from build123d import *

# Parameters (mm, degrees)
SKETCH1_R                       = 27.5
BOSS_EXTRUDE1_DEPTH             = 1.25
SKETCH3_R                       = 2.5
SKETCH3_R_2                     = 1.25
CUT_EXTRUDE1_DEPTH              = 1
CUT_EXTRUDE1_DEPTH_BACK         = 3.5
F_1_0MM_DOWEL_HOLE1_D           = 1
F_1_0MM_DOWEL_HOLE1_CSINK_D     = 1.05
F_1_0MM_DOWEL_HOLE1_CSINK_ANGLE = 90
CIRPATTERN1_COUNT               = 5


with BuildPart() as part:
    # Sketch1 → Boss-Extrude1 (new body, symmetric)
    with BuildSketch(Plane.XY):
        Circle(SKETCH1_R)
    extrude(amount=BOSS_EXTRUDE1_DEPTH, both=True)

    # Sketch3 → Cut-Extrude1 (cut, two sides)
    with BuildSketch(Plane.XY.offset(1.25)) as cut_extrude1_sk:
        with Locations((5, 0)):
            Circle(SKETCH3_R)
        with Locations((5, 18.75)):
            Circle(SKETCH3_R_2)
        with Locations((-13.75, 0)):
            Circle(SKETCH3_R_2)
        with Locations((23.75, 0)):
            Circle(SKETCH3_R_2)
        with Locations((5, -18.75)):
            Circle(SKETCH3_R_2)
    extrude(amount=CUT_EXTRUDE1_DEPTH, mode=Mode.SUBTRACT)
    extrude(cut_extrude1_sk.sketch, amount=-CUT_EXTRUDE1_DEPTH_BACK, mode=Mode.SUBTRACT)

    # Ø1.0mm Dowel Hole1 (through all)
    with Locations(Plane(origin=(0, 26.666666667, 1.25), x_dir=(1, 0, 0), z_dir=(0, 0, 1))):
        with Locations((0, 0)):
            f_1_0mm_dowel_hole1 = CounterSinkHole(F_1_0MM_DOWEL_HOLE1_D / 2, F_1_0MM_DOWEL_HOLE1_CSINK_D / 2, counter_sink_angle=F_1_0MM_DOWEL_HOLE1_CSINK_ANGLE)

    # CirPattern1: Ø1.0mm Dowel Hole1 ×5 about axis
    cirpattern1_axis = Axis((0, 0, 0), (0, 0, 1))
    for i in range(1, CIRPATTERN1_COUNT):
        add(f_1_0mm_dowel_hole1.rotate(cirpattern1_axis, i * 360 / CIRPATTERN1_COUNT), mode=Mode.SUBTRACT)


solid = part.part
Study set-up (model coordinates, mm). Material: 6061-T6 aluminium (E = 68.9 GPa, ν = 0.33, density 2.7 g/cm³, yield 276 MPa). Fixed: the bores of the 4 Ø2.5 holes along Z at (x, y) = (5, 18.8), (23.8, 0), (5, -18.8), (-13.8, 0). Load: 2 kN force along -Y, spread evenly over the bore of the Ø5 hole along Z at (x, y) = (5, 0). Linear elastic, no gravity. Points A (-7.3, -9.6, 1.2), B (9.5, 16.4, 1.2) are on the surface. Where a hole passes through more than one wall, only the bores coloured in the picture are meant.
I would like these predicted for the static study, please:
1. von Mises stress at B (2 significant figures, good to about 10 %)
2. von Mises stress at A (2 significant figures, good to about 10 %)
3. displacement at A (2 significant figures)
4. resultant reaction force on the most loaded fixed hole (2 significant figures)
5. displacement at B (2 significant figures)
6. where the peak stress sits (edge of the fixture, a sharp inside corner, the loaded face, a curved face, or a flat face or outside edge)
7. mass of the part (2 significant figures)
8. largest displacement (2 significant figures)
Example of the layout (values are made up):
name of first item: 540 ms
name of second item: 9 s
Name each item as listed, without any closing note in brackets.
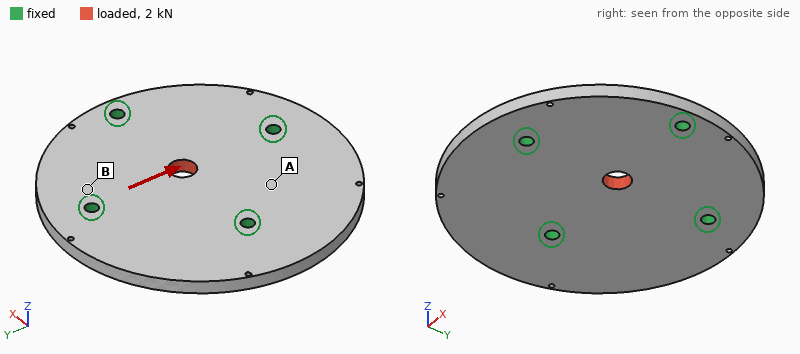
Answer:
von Mises stress at B: 13 MPa
von Mises stress at A: 6.8 MPa
displacement at A: 2.3 µm
resultant reaction force on the most loaded fixed hole: 650 N
displacement at B: 2.1 µm
where the peak stress sits: the loaded face
mass of the part: 16 g
largest displacement: 8.2 µm
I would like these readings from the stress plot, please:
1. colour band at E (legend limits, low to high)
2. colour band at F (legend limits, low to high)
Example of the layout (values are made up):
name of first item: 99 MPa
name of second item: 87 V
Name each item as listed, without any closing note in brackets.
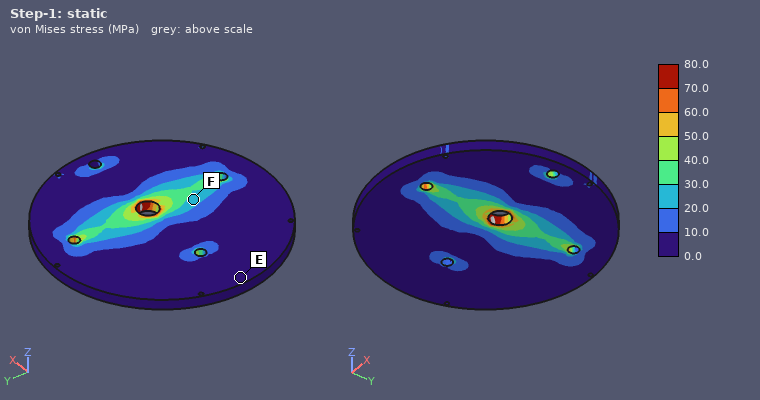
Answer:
colour band at E: 0.0 to 10.0 MPa
colour band at F: 20.0 to 30.0 MPa
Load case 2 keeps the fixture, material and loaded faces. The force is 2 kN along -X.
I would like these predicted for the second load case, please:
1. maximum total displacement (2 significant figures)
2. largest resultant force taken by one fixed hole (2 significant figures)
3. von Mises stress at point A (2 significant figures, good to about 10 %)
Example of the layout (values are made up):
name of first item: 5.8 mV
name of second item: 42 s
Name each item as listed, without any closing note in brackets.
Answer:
maximum total displacement: 8.1 µm
largest resultant force taken by one fixed hole: 670 N
von Mises stress at point A: 8.2 MPa
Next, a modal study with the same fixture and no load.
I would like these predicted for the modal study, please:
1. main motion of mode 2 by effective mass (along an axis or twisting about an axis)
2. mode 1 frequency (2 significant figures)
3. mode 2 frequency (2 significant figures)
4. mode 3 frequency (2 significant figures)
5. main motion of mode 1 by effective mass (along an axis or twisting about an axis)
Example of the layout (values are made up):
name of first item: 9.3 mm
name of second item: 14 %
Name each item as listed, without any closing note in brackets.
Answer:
main motion of mode 2 by effective mass: along Z
mode 1 frequency: 6600 Hz
mode 2 frequency: 7400 Hz
mode 3 frequency: 11 kHz
main motion of mode 1 by effective mass: twisting about X
